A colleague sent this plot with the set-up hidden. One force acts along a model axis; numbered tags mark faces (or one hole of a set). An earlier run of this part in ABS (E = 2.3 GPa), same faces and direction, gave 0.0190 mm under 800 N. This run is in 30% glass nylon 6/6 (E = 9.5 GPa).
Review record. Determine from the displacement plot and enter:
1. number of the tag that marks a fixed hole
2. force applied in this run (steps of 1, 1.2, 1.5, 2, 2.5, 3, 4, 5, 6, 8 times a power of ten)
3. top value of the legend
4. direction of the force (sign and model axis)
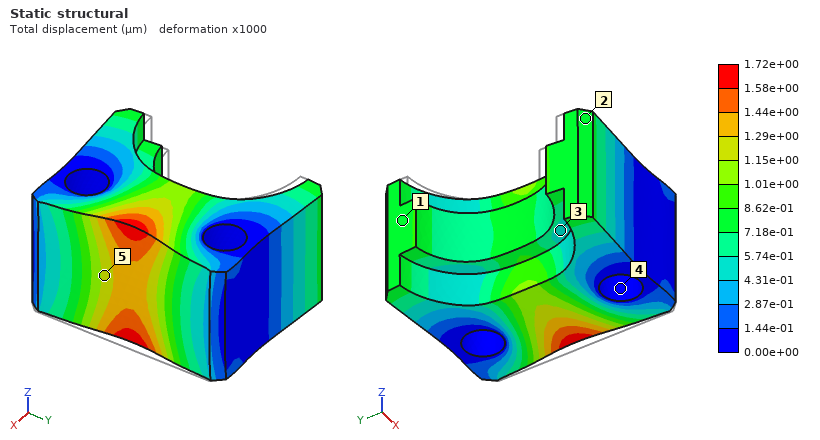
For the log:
4
300 N
1.72e+00 µm
-X
